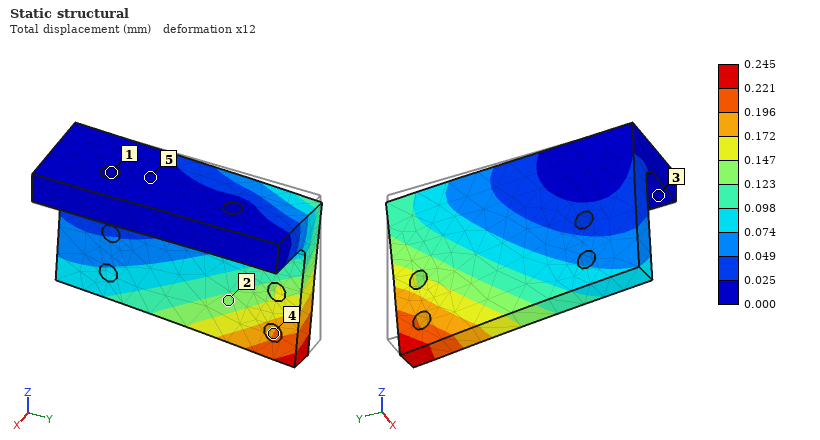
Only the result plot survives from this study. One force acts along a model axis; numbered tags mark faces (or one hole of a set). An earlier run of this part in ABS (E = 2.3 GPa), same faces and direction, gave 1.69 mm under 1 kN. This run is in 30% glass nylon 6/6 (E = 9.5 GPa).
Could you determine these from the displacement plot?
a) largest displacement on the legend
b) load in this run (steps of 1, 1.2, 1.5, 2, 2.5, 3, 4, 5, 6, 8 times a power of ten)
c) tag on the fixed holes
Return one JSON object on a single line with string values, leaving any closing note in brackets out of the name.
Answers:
{"largest displacement on the legend": "0.245 mm", "load in this run": "600 N", "tag on the fixed holes": "1"}
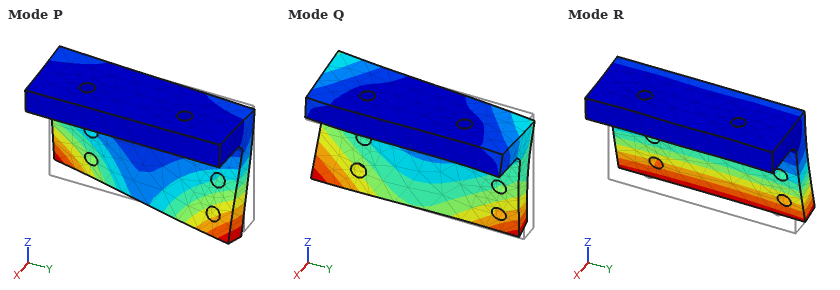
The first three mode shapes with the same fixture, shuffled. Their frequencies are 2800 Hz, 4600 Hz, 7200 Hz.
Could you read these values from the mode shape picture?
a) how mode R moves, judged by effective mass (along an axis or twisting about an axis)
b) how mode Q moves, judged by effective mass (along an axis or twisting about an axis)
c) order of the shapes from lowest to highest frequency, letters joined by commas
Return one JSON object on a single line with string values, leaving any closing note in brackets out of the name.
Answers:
{"how mode R moves, judged by effective mass": "along X", "how mode Q moves, judged by effective mass": "along Y", "order of the shapes from lowest to highest frequency, letters joined by commas": "R, P, Q"}
